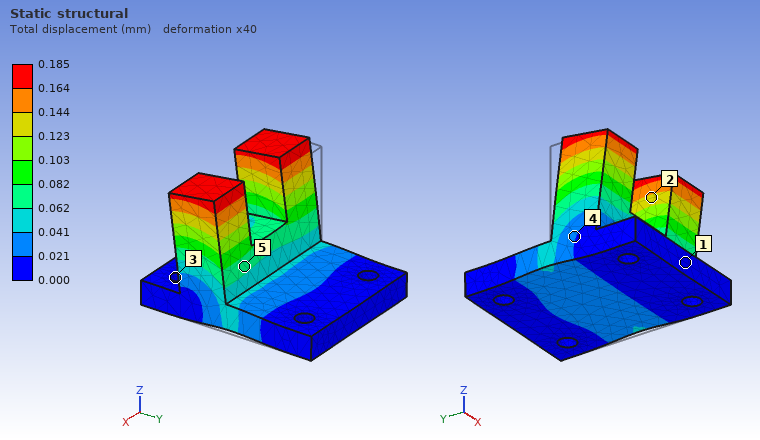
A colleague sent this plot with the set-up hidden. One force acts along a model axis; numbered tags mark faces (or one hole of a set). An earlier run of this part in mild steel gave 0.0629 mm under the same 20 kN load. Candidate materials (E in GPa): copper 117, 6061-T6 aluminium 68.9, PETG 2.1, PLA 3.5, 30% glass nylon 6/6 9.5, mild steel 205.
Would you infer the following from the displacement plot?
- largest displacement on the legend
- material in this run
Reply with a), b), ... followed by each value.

a) 0.185 mm
b) 6061-T6 aluminium
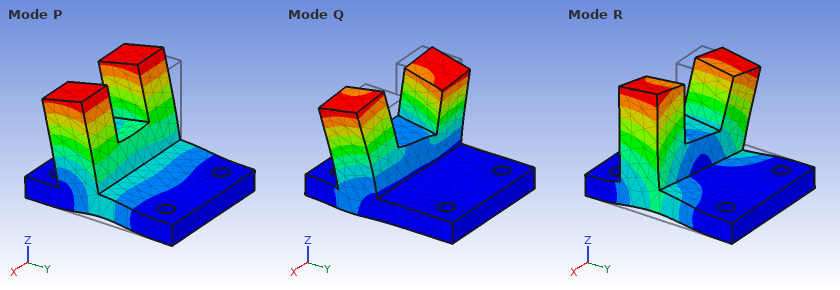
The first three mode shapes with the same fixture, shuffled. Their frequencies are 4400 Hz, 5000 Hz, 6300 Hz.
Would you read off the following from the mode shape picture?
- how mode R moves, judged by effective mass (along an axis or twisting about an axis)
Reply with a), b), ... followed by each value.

a) along X
